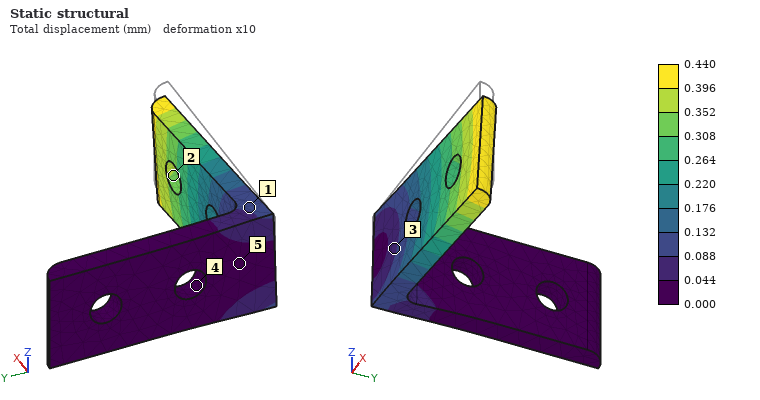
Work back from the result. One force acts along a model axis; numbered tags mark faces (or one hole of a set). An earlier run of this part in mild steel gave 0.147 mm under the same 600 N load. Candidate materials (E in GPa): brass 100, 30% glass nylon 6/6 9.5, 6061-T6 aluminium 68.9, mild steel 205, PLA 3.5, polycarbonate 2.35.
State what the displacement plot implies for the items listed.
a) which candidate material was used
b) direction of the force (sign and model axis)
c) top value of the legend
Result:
6061-T6 aluminium
-Z
0.440 mm
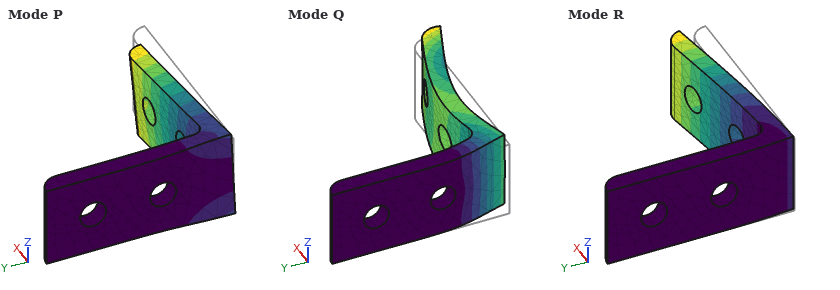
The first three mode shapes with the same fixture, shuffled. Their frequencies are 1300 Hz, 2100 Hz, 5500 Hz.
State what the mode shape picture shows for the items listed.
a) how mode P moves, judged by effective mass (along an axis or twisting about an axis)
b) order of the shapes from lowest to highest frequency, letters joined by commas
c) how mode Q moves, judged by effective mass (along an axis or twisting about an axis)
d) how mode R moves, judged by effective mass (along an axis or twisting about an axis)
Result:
along Z
R, P, Q
along X
along Y
